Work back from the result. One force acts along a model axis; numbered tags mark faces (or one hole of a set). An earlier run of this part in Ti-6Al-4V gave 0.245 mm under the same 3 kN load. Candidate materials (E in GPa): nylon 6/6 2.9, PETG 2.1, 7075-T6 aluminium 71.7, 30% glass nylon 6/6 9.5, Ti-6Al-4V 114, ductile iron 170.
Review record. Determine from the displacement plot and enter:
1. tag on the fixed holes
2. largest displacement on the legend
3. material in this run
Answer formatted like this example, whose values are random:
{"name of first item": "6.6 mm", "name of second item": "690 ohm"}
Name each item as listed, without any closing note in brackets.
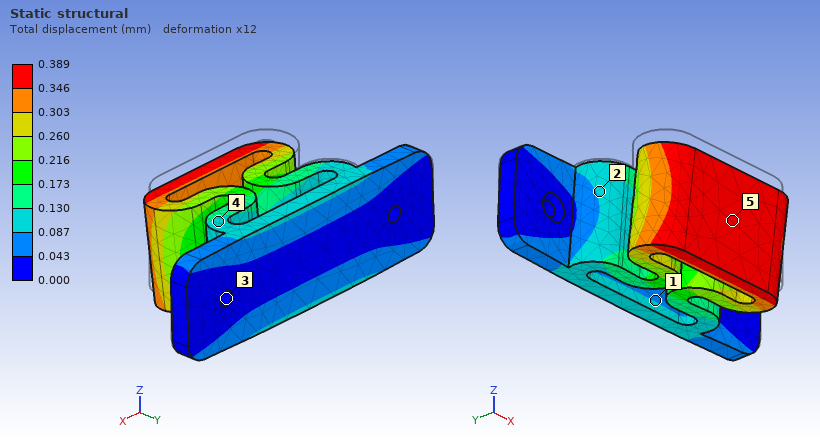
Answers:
{"tag on the fixed holes": "3", "largest displacement on the legend": "0.389 mm", "material in this run": "7075-T6 aluminium"}
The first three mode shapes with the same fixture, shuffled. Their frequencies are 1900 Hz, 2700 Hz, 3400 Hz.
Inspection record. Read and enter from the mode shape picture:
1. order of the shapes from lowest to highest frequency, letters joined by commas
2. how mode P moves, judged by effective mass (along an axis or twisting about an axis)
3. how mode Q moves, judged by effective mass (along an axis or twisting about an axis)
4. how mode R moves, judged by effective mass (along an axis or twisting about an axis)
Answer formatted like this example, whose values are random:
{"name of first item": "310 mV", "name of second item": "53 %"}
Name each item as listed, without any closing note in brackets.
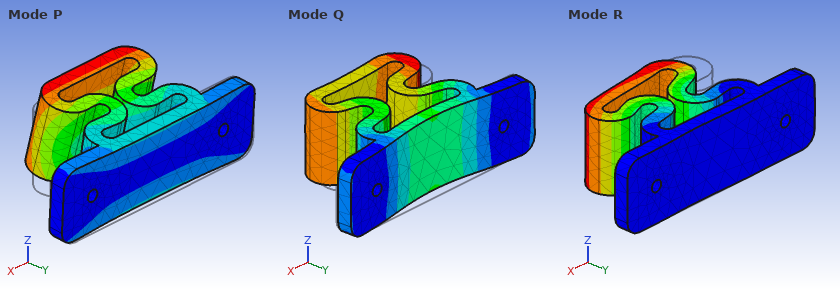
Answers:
{"order of the shapes from lowest to highest frequency, letters joined by commas": "P, R, Q", "how mode P moves, judged by effective mass": "along Z", "how mode Q moves, judged by effective mass": "along Y", "how mode R moves, judged by effective mass": "along X"}
